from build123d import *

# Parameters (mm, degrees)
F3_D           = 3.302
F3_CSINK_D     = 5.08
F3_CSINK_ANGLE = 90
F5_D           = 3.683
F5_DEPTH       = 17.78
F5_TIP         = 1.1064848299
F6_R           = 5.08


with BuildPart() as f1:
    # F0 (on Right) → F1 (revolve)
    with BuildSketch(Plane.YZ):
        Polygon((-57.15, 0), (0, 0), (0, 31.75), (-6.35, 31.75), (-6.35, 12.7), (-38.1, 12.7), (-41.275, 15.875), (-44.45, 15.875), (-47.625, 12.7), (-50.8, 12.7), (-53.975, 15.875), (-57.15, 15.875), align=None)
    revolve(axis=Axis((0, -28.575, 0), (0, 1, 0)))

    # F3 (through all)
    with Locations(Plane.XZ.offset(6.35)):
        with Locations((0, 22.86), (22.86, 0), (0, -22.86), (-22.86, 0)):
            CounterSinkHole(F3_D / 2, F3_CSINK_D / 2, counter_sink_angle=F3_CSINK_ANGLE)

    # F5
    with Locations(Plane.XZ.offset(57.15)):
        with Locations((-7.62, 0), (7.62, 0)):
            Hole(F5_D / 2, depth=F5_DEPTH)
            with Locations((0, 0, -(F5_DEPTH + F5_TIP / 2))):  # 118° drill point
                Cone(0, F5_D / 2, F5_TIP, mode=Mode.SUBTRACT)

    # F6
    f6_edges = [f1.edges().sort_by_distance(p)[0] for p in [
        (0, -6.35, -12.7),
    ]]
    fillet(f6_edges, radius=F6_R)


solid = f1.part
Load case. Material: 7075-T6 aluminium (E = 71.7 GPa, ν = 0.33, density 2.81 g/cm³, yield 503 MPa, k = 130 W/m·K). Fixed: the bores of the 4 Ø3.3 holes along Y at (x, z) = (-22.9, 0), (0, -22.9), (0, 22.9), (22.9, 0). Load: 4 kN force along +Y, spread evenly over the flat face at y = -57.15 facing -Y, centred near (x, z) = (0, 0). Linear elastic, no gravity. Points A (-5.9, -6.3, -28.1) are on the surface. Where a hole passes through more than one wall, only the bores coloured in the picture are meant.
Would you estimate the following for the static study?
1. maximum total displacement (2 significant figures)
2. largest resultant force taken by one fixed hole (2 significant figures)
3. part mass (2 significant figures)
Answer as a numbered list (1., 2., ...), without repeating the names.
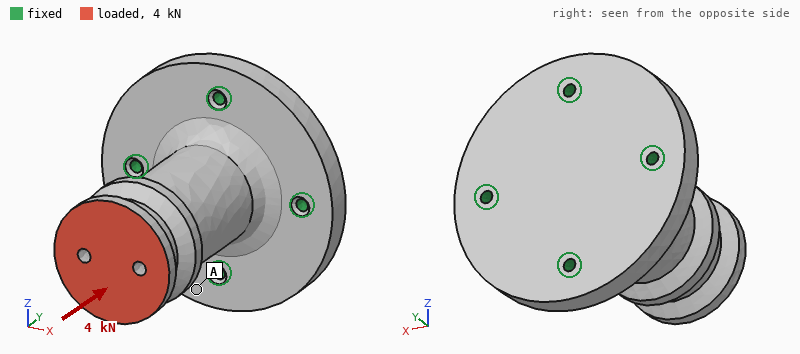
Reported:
1. 15 µm
2. 1.1 kN
3. 140 g
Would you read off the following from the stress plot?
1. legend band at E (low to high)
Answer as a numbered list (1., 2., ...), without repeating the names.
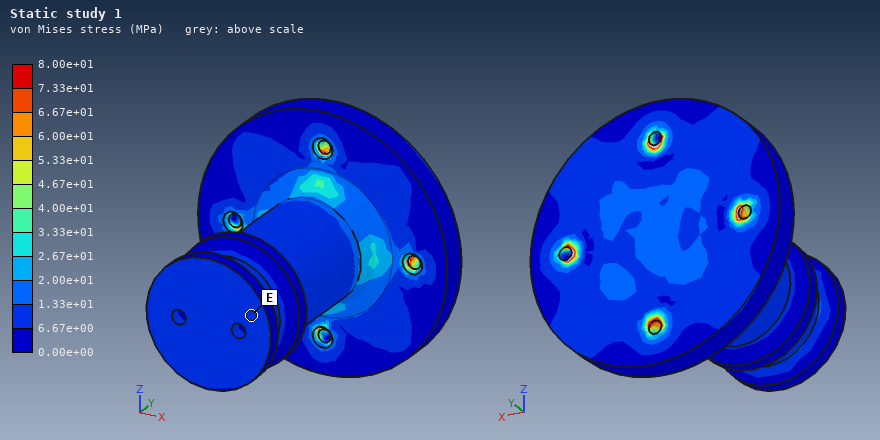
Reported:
1. 6.67e+00 to 1.33e+01 MPa
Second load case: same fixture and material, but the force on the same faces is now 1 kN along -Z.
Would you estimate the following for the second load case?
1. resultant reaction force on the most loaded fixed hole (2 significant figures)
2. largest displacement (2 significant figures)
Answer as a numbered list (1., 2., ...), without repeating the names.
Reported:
1. 1.3 kN
2. 67 µm
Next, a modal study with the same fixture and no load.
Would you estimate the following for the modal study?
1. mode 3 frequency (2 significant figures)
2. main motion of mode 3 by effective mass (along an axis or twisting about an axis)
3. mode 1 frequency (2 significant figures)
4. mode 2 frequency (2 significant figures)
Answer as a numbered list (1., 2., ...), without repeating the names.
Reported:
1. 9800 Hz
2. along Y
3. 3800 Hz
4. 3800 Hz
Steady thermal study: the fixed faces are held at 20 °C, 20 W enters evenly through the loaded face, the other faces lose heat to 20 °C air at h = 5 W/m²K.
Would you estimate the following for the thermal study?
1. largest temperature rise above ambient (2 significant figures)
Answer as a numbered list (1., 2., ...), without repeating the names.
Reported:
1. 19 K
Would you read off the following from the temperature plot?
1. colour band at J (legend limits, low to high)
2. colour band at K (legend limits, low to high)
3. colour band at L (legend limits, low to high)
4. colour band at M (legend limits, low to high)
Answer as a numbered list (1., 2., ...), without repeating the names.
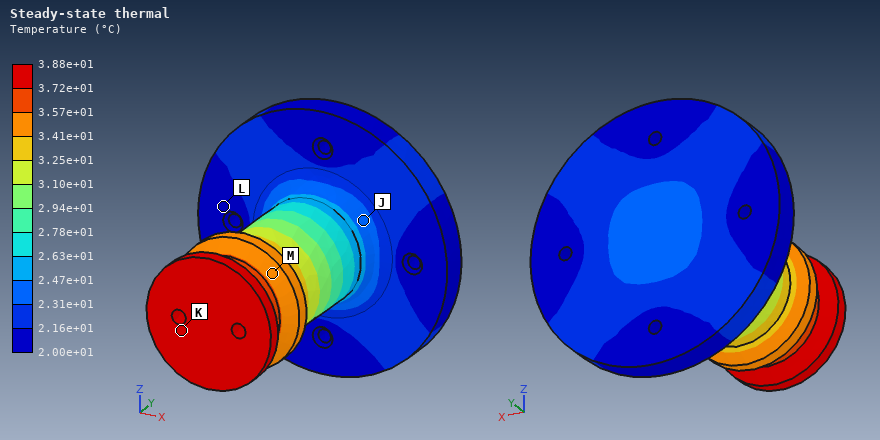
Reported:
1. 2.31e+01 to 2.47e+01 °C
2. 3.72e+01 to 3.88e+01 °C
3. 2.00e+01 to 2.16e+01 °C
4. 3.41e+01 to 3.57e+01 °C
